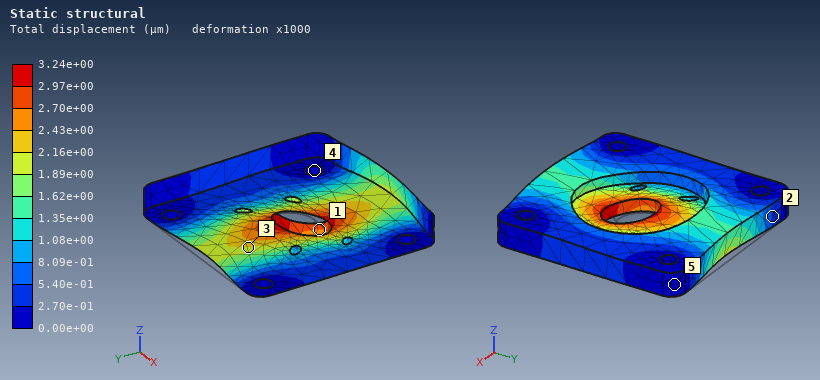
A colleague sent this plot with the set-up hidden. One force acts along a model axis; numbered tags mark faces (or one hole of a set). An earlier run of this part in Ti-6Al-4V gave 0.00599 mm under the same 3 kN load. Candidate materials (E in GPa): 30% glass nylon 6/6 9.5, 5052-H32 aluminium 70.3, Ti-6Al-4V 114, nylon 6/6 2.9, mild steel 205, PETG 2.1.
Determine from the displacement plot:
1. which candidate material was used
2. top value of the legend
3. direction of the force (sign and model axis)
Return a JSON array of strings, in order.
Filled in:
["mild steel", "3.24e+00 µm", "-Y"]
